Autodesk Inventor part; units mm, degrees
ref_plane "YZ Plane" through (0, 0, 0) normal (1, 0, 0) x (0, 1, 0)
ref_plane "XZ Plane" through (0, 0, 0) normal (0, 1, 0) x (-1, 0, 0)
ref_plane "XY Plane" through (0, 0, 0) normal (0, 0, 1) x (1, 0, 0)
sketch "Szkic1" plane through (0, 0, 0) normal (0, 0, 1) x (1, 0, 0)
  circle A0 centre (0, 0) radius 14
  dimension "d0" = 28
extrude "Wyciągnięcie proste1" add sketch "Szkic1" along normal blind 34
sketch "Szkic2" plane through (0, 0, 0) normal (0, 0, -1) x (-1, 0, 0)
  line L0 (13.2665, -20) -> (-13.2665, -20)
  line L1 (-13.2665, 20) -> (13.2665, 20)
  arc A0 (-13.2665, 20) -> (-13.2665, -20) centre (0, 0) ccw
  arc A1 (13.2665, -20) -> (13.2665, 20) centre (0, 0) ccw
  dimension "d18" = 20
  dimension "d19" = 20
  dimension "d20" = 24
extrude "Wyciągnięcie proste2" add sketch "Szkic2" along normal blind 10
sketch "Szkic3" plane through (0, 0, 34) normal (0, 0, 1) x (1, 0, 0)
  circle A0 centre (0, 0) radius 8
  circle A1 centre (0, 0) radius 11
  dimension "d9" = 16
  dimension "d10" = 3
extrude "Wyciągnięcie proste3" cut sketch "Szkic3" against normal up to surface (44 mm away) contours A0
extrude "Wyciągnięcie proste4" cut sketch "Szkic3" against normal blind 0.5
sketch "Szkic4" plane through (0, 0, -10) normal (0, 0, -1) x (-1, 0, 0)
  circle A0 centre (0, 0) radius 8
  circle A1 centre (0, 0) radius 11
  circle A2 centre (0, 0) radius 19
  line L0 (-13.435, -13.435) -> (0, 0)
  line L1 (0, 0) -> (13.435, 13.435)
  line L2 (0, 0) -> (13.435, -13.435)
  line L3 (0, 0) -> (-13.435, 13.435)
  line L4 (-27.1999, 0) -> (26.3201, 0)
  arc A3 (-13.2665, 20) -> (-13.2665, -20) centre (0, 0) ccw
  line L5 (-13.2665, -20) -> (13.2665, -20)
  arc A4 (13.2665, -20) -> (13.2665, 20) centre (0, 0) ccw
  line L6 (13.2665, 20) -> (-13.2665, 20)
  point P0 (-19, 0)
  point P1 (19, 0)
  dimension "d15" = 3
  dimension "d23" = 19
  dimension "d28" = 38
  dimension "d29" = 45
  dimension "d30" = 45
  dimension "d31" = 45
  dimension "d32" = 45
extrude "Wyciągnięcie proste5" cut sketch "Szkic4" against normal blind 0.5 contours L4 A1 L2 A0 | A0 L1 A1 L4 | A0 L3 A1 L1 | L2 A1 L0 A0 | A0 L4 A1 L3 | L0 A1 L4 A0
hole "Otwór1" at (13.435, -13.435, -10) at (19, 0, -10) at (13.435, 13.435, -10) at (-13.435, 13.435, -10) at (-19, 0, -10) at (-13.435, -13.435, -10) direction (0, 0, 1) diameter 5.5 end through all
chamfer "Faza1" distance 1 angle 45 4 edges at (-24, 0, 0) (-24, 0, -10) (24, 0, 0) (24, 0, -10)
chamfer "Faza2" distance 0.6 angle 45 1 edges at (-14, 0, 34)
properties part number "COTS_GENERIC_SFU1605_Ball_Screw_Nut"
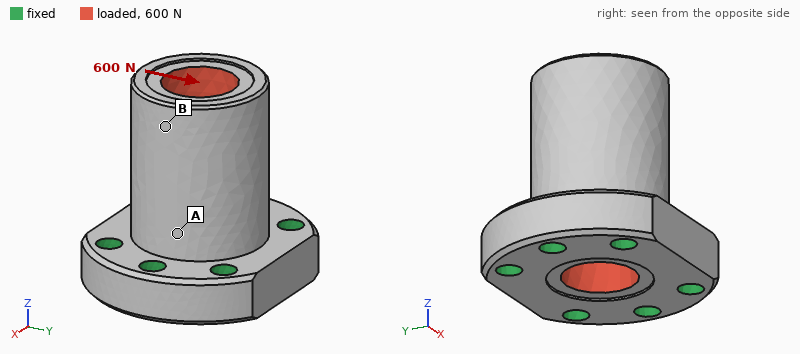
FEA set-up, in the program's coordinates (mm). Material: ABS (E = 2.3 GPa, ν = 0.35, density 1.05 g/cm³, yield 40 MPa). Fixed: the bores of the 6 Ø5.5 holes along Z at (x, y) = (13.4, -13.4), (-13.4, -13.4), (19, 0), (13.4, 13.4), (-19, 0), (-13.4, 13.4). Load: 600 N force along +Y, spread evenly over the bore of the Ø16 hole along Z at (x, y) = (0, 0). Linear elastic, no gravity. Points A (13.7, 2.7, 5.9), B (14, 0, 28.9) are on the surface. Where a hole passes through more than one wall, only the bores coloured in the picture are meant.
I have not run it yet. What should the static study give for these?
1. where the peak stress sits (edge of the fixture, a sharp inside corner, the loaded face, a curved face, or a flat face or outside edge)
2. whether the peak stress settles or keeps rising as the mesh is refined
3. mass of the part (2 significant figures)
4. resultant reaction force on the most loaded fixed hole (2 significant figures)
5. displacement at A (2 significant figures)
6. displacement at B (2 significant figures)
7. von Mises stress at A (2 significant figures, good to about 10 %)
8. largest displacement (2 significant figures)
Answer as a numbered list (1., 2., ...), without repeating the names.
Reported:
1. edge of the fixture
2. keeps rising
3. 28 g
4. 230 N
5. 0.026 mm
6. 0.10 mm
7. 2.0 MPa
8. 0.13 mm
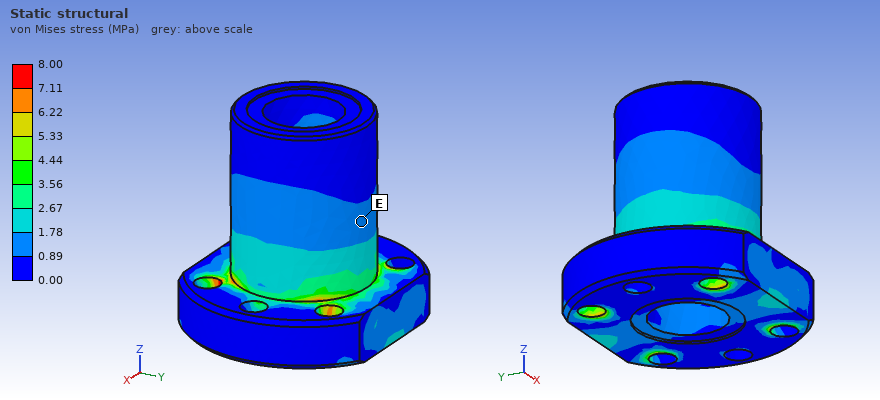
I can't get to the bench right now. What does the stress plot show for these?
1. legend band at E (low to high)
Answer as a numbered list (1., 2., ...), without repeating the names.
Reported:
1. 0.89 to 1.78 MPa
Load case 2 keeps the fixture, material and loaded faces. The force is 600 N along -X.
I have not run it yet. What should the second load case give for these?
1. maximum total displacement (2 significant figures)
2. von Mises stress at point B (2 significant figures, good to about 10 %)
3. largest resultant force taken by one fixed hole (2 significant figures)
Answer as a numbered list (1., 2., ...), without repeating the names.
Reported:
1. 0.11 mm
2. 0.47 MPa
3. 200 N
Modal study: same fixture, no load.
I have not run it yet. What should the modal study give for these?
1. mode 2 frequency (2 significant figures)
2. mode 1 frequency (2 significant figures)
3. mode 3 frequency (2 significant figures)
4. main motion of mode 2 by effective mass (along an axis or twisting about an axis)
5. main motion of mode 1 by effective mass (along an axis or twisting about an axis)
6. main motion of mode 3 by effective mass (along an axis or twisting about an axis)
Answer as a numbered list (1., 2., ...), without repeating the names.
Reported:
1. 3200 Hz
2. 3000 Hz
3. 6100 Hz
4. along X
5. along Y
6. twisting about Z
